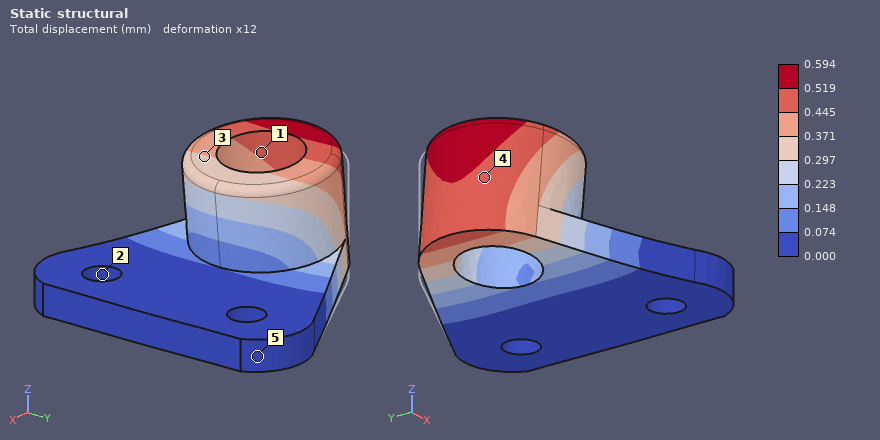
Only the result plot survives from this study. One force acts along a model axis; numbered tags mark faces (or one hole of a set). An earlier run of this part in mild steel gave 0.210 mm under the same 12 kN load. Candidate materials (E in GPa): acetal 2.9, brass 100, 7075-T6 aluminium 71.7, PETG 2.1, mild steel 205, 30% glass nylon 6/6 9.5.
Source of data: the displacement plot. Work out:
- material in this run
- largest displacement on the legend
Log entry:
7075-T6 aluminium
0.594 mm
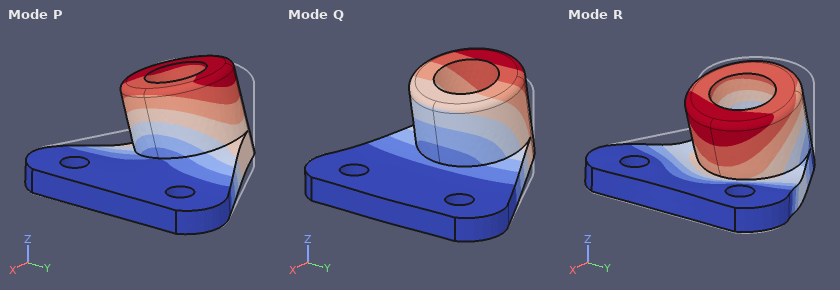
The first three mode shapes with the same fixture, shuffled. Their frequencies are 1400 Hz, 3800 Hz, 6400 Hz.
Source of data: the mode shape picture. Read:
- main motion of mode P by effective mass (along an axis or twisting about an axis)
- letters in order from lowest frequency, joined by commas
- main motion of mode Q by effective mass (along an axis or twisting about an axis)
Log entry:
along Y
Q, P, R
along Z
